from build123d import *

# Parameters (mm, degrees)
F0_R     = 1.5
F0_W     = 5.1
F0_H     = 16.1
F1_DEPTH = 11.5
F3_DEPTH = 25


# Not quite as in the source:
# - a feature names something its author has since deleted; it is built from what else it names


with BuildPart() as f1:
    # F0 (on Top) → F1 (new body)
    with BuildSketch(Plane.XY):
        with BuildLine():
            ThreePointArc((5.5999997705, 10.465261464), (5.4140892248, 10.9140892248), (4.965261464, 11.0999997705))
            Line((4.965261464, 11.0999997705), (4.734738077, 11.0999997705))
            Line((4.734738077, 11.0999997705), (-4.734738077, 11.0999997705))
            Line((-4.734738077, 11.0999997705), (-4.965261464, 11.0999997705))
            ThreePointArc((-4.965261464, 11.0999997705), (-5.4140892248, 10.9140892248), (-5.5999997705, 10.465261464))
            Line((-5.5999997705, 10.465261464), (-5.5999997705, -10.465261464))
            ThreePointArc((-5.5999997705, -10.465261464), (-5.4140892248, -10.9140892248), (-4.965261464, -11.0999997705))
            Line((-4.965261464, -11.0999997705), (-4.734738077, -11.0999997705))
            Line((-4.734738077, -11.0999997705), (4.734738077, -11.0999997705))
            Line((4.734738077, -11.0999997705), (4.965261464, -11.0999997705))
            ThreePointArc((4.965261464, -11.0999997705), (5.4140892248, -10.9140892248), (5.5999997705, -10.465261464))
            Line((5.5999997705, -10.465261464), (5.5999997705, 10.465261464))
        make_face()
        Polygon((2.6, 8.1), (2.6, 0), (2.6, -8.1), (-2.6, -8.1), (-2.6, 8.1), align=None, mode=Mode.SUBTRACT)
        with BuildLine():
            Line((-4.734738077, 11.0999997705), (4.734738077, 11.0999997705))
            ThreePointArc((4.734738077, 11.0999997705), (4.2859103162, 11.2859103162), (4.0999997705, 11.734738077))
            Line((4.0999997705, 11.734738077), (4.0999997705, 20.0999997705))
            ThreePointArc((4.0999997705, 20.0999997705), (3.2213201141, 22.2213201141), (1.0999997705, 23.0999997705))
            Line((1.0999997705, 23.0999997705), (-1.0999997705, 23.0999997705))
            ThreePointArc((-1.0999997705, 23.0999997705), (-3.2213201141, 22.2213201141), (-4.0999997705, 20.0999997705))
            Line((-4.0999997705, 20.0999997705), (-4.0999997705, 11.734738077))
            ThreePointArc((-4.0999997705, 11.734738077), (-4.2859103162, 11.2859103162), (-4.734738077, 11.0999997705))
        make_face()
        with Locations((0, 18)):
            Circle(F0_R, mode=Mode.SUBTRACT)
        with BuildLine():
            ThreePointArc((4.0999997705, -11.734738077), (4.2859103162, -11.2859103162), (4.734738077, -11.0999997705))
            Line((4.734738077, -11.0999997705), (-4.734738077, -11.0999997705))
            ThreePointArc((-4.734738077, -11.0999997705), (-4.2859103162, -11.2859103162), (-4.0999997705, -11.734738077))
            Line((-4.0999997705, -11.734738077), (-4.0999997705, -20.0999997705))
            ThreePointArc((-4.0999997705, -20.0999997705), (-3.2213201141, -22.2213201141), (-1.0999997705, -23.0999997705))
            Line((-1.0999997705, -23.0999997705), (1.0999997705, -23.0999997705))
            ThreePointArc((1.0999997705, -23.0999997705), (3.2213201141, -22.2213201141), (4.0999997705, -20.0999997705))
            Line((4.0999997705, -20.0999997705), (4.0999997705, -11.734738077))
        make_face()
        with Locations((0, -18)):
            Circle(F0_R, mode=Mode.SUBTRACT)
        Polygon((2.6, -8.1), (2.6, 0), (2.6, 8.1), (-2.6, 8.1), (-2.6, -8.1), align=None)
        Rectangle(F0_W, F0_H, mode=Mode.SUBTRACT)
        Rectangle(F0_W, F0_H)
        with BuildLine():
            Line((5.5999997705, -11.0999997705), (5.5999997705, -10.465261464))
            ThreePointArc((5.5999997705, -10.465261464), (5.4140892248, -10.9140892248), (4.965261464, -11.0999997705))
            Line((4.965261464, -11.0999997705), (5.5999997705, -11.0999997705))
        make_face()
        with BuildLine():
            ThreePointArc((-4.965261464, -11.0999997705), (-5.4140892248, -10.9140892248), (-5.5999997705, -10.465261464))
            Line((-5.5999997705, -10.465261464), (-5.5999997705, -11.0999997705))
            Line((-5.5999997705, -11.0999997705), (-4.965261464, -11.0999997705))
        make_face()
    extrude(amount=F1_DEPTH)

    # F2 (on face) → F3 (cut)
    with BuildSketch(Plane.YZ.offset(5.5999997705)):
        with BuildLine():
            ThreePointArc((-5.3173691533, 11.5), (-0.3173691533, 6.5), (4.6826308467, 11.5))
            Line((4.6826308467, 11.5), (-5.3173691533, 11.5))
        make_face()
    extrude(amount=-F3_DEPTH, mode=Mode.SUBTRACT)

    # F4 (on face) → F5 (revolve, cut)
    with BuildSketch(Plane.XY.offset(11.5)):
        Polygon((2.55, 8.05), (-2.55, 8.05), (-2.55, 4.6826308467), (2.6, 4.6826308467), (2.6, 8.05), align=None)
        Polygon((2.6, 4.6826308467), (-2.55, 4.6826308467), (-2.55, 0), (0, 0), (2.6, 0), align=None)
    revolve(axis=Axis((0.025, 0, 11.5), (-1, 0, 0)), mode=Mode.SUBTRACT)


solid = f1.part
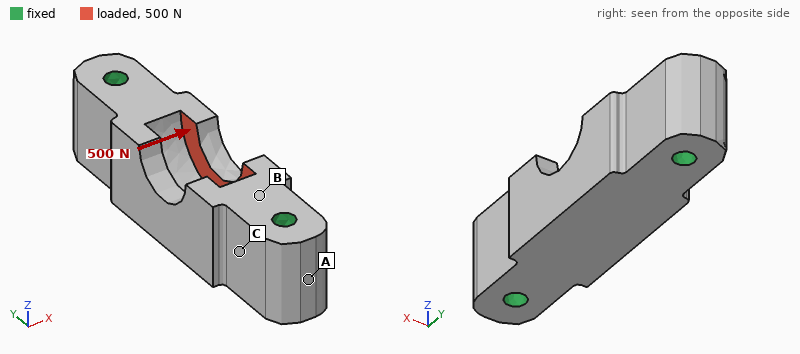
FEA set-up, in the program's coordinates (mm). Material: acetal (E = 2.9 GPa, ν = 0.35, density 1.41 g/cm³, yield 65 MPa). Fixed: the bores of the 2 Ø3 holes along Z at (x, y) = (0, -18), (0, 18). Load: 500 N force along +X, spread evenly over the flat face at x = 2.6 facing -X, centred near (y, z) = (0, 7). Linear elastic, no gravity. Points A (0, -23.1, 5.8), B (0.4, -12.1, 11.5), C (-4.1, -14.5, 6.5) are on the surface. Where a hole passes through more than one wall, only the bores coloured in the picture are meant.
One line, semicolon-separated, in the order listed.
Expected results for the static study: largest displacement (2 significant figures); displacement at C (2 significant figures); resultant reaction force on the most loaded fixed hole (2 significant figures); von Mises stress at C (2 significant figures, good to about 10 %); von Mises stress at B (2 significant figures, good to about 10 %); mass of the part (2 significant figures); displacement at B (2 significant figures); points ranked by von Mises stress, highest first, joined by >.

0.21 mm; 0.031 mm; 260 N; 5.8 MPa; 10 MPa; 5.8 g; 0.046 mm; B > C > A
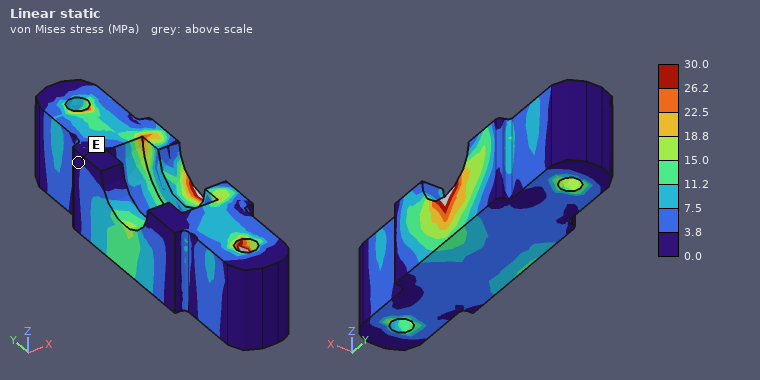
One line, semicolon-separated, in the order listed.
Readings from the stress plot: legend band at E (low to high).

0.0 to 3.8 MPa
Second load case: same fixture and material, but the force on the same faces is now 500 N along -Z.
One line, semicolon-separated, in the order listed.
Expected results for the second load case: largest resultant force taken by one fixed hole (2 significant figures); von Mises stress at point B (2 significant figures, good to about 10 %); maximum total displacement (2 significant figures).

290 N; 8.6 MPa; 0.13 mm
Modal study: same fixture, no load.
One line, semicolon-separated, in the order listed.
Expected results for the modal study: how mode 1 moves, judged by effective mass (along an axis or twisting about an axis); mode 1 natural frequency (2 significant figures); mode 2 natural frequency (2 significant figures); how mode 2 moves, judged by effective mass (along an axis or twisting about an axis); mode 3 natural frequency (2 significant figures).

along X; 7100 Hz; 8700 Hz; along Z; 11 kHz
